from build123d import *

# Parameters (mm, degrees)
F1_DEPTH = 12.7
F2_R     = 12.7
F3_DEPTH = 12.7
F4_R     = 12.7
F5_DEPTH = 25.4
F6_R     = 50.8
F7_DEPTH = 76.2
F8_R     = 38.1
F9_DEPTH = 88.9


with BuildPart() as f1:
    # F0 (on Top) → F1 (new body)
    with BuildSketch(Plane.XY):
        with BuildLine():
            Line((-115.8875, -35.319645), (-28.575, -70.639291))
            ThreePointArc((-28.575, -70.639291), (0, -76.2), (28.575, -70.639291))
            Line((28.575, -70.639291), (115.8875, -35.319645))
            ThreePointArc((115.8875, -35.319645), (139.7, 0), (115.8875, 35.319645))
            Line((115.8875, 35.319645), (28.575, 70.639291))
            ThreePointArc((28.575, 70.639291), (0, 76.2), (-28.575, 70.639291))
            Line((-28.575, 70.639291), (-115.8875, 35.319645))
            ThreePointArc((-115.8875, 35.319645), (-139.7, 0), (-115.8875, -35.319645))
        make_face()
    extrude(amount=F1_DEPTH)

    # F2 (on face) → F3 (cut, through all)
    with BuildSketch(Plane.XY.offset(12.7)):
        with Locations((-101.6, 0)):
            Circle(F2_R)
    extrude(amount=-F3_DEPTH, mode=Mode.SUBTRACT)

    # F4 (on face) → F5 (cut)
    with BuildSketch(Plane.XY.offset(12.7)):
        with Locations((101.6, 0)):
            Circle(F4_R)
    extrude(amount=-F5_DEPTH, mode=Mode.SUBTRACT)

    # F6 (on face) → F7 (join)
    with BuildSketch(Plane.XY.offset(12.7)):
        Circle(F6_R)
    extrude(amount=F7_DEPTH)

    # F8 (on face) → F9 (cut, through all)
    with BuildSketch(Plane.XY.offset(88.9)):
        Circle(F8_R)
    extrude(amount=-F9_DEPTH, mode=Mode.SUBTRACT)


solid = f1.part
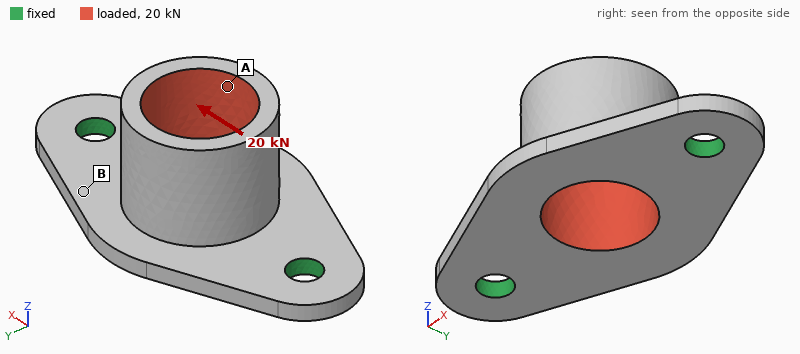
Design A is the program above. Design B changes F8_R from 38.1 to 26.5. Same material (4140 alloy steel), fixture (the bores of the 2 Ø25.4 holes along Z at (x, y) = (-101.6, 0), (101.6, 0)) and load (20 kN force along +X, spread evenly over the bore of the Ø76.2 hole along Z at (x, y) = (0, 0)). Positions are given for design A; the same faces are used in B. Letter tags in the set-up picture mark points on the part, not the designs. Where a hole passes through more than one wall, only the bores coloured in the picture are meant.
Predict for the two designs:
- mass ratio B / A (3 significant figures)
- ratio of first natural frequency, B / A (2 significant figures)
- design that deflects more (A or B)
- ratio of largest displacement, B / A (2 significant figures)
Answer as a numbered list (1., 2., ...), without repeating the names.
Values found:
1. 1.37
2. 0.86
3. A
4. 0.85
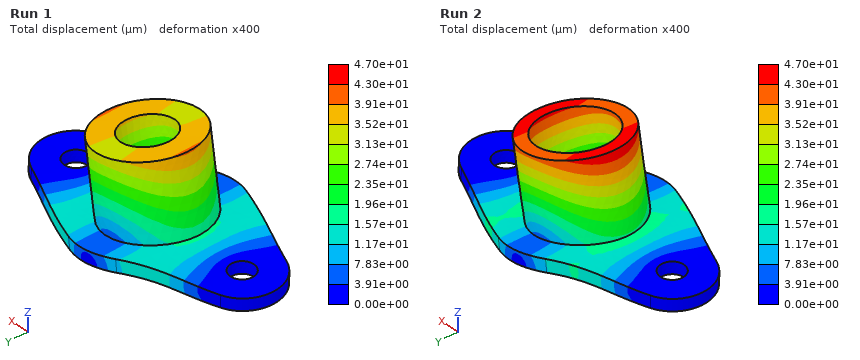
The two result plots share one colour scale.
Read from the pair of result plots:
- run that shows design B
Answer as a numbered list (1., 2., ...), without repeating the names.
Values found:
1. Run 1
